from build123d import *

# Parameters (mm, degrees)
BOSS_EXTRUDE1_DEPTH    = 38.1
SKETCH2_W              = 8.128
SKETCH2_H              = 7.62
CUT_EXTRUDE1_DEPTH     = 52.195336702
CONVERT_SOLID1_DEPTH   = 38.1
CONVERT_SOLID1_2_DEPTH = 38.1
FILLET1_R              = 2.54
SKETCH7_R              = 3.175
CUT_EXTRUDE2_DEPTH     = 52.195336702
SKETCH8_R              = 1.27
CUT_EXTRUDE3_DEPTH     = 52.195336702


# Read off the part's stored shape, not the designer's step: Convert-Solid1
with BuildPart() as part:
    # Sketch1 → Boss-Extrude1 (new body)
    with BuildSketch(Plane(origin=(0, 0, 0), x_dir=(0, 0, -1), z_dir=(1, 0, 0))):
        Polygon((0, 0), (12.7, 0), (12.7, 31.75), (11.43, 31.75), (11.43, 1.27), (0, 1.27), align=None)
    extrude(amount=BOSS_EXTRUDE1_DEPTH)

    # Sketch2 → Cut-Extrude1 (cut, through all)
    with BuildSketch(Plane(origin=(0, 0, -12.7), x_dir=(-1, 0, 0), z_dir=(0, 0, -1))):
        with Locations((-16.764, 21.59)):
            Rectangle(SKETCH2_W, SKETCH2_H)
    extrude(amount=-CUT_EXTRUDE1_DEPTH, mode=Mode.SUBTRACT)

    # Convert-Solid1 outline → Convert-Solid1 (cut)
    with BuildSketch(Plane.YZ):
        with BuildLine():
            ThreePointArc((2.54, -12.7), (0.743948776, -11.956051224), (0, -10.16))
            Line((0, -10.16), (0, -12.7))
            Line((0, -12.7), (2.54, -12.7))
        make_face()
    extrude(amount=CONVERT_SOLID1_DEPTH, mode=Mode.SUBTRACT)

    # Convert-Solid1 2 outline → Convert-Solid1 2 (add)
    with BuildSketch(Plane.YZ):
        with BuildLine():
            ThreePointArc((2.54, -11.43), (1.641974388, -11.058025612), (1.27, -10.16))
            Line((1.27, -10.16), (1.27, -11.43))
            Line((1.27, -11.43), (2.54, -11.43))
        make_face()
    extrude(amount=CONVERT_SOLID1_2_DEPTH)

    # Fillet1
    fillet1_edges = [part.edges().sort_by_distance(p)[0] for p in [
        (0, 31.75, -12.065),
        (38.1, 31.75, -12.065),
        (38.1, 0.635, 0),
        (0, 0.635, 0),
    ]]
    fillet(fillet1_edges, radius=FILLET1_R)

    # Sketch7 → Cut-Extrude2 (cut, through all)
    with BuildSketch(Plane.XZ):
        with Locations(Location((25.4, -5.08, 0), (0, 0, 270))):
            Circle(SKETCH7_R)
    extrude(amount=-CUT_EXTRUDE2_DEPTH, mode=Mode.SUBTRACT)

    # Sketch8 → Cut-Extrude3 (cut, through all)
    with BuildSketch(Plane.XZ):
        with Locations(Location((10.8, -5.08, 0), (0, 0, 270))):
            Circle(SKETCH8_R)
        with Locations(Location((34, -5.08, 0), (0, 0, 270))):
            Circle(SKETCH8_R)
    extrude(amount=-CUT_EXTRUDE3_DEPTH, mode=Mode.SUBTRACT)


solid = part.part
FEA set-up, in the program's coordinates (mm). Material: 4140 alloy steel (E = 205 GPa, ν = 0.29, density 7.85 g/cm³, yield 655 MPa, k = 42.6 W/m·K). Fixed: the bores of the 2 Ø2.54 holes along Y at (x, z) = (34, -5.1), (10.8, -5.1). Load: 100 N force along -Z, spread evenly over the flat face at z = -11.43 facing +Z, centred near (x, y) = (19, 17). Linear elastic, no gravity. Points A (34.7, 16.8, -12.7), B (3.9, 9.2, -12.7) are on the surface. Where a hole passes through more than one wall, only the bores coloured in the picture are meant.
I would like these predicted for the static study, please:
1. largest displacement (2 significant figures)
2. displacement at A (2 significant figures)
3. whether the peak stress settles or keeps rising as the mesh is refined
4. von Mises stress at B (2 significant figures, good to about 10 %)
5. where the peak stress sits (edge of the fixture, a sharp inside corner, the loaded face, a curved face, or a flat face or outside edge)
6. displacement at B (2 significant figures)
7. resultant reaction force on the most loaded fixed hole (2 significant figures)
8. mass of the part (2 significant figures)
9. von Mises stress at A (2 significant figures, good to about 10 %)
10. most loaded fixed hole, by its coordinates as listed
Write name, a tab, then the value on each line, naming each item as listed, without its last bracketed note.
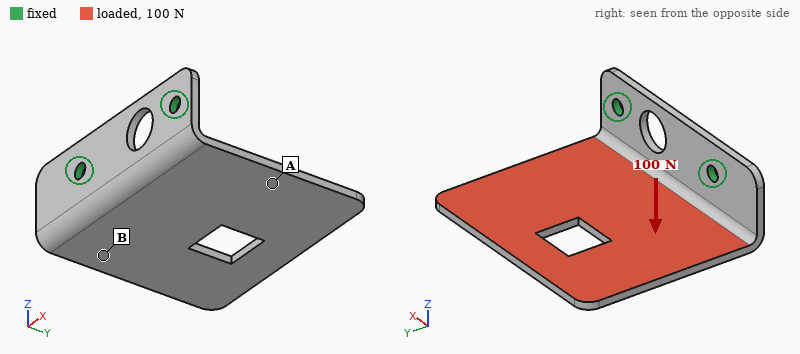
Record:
largest displacement	0.56 mm
displacement at A	0.25 mm
whether the peak stress settles or keeps rising as the mesh is refined	keeps rising
von Mises stress at B	78 MPa
where the peak stress sits	edge of the fixture
displacement at B	0.12 mm
resultant reaction force on the most loaded fixed hole	64 N
mass of the part	15 g
von Mises stress at A	40 MPa
most loaded fixed hole, by its coordinates as listed	(10.8, -5.1)
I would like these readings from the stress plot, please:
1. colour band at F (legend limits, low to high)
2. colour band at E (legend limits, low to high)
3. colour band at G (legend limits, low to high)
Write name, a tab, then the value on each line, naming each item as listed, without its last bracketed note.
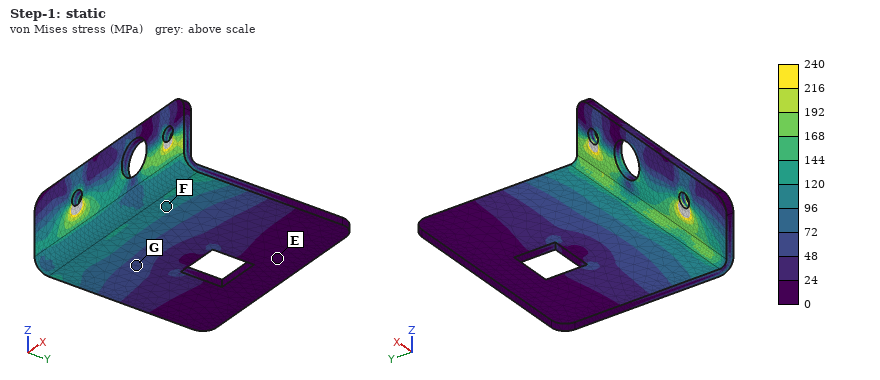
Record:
colour band at F	96 to 120 MPa
colour band at E	0 to 24 MPa
colour band at G	48 to 72 MPa
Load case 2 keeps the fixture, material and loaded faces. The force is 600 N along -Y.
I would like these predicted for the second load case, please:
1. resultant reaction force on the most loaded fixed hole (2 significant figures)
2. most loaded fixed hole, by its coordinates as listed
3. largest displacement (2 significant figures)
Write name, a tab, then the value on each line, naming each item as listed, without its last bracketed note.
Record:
resultant reaction force on the most loaded fixed hole	380 N
most loaded fixed hole, by its coordinates as listed	(10.8, -5.1)
largest displacement	0.27 mm
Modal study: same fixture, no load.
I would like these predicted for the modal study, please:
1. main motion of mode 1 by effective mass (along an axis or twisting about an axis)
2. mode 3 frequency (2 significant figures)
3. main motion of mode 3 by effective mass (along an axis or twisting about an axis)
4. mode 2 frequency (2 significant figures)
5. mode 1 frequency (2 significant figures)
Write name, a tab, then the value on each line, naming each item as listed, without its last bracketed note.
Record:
main motion of mode 1 by effective mass	along Z
mode 3 frequency	3500 Hz
main motion of mode 3 by effective mass	along X
mode 2 frequency	1900 Hz
mode 1 frequency	810 Hz
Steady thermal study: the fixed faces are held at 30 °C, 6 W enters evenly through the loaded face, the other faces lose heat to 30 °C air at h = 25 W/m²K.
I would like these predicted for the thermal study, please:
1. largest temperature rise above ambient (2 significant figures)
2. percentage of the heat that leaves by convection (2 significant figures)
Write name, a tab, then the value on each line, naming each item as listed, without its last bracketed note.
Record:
largest temperature rise above ambient	59 K
percentage of the heat that leaves by convection	29 %
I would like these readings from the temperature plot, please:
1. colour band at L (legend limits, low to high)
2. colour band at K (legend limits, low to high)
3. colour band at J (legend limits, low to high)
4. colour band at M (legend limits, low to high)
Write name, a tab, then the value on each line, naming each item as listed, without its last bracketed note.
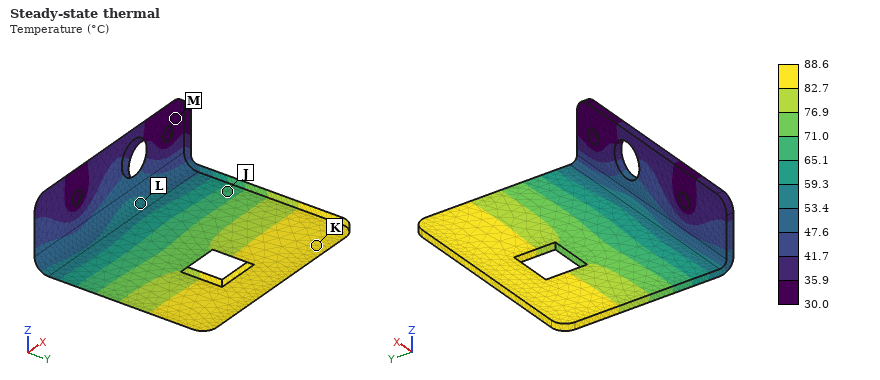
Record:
colour band at L	53.4 to 59.3 °C
colour band at K	82.7 to 88.6 °C
colour band at J	65.1 to 71.0 °C
colour band at M	30.0 to 35.9 °C
